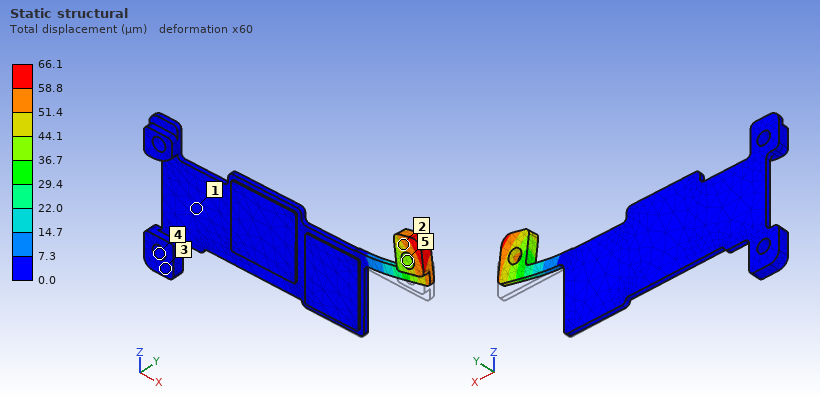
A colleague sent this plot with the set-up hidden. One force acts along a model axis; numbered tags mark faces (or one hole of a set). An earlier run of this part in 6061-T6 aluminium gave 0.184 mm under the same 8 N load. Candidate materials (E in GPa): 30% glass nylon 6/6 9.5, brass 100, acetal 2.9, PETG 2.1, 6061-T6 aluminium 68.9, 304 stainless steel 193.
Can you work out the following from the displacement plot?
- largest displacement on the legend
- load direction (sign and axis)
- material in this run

66.1 µm
+Z
304 stainless steel
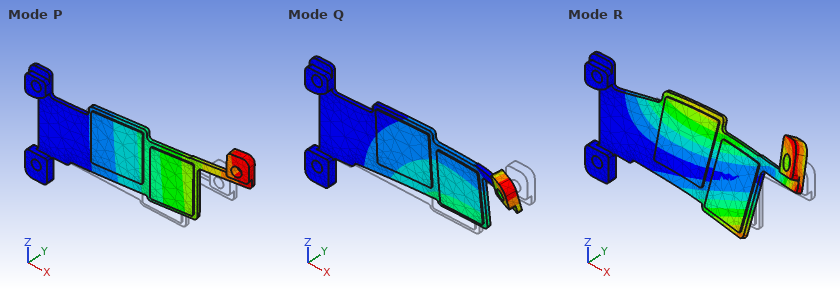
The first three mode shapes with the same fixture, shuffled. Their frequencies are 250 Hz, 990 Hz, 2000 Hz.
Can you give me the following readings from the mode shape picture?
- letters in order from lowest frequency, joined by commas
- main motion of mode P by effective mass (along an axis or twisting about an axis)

P, Q, R
along Y
